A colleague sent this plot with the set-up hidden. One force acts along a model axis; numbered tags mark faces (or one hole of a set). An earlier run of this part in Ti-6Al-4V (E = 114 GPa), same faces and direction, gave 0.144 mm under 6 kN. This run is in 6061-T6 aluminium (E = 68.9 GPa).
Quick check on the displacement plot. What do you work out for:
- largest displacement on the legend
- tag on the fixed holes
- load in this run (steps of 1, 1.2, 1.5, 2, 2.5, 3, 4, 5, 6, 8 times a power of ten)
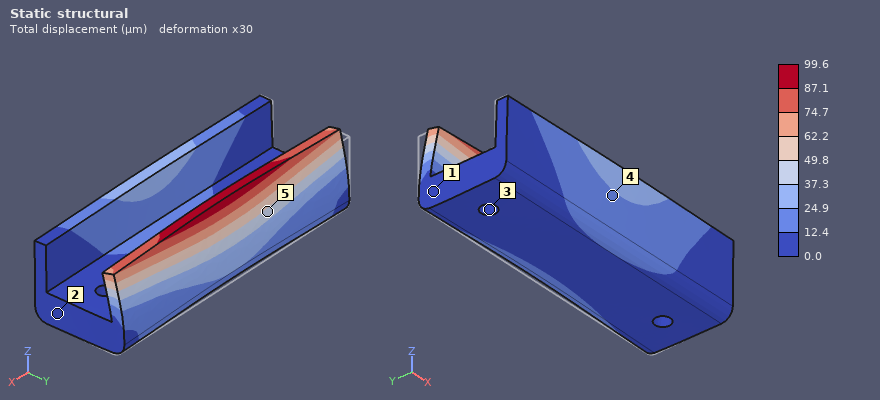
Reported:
99.6 µm
3
2.5 kN
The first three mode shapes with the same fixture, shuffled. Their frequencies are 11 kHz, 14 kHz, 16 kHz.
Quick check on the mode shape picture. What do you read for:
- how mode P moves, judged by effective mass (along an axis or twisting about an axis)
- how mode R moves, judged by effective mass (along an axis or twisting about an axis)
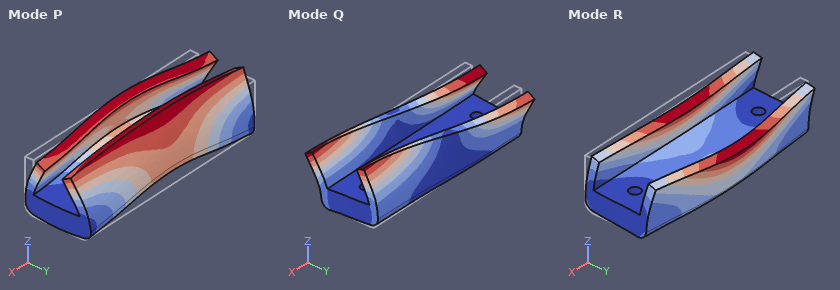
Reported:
along Z
along Y
